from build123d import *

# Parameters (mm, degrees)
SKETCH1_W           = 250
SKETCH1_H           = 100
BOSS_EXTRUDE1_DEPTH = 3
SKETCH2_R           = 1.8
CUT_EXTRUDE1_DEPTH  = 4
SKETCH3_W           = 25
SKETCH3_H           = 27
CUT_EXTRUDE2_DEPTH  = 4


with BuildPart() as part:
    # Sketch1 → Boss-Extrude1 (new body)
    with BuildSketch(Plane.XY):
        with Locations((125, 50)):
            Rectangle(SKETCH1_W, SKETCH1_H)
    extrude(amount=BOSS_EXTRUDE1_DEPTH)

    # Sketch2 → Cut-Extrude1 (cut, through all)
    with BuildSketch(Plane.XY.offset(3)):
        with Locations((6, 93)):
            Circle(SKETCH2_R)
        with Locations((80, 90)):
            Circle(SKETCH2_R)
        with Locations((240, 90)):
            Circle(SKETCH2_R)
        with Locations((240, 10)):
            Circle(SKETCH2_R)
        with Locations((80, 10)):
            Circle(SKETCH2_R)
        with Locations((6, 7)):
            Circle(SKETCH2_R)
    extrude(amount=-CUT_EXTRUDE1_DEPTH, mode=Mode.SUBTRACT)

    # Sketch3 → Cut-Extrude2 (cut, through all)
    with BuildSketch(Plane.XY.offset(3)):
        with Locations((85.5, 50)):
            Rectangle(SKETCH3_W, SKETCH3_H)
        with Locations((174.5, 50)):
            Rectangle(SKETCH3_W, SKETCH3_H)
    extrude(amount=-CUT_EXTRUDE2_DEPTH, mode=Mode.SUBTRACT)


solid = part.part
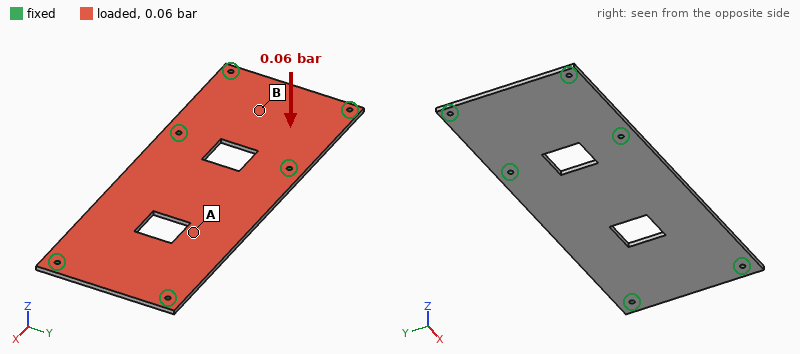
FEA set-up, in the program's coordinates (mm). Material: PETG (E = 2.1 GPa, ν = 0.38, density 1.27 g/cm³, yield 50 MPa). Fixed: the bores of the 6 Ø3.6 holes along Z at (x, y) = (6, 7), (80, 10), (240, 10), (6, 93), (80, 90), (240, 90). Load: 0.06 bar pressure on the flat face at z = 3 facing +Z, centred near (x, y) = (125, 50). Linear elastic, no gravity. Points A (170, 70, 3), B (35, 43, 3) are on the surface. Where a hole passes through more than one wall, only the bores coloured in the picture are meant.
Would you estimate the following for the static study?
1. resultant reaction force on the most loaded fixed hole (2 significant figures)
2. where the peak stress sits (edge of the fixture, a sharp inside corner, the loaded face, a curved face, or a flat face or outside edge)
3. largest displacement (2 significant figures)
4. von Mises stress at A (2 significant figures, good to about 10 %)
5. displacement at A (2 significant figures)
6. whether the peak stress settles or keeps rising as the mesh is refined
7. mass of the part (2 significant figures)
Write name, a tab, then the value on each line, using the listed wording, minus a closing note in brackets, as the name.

resultant reaction force on the most loaded fixed hole	34 N
where the peak stress sits	edge of the fixture
largest displacement	3.0 mm
von Mises stress at A	5.7 MPa
displacement at A	2.8 mm
whether the peak stress settles or keeps rising as the mesh is refined	keeps rising
mass of the part	90 g
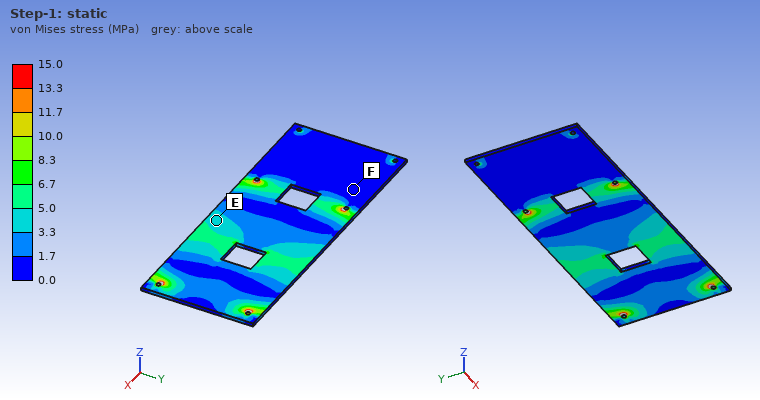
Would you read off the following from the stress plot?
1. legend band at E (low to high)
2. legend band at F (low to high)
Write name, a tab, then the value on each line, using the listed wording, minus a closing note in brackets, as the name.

legend band at E	3.3 to 5.0 MPa
legend band at F	0.0 to 1.7 MPa
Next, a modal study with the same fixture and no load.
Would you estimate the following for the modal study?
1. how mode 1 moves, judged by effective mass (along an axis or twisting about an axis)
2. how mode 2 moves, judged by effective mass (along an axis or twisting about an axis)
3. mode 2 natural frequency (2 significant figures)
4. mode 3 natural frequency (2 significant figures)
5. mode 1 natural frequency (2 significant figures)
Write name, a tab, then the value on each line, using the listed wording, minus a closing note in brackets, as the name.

how mode 1 moves, judged by effective mass	along Z
how mode 2 moves, judged by effective mass	twisting about X
mode 2 natural frequency	220 Hz
mode 3 natural frequency	370 Hz
mode 1 natural frequency	140 Hz
